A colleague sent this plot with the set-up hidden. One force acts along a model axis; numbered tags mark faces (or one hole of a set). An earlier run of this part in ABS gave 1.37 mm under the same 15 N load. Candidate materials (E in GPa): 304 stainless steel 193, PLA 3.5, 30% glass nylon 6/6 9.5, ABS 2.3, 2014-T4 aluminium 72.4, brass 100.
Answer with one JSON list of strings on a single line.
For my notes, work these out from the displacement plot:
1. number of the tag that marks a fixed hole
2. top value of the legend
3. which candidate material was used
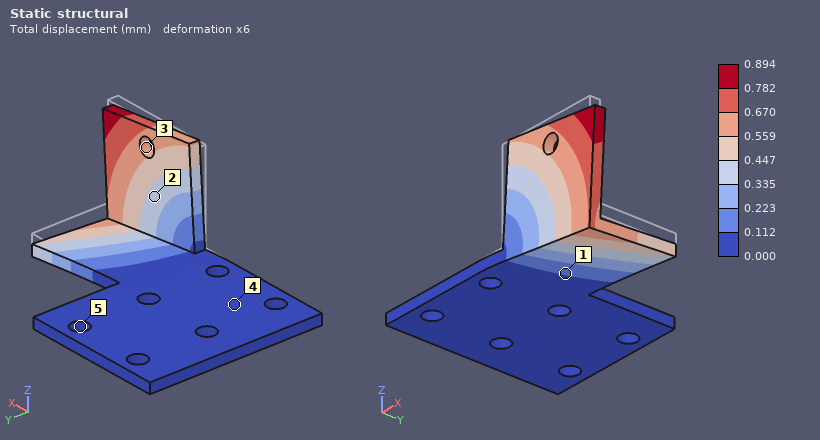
["5", "0.894 mm", "PLA"]
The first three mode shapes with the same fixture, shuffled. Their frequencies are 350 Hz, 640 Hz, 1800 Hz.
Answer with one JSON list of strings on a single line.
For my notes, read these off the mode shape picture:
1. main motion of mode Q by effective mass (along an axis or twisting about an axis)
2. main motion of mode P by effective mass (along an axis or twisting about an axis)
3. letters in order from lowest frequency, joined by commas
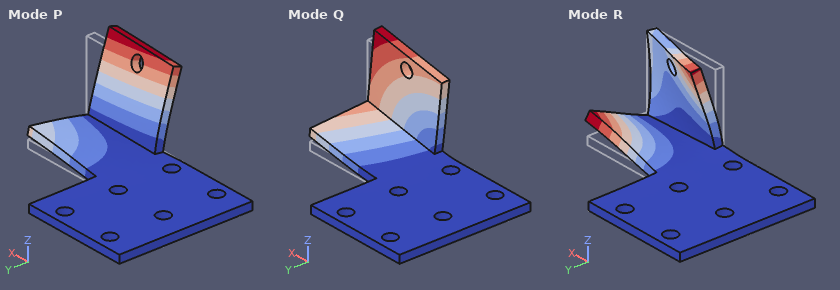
["along Z", "along Y", "Q, P, R"]
